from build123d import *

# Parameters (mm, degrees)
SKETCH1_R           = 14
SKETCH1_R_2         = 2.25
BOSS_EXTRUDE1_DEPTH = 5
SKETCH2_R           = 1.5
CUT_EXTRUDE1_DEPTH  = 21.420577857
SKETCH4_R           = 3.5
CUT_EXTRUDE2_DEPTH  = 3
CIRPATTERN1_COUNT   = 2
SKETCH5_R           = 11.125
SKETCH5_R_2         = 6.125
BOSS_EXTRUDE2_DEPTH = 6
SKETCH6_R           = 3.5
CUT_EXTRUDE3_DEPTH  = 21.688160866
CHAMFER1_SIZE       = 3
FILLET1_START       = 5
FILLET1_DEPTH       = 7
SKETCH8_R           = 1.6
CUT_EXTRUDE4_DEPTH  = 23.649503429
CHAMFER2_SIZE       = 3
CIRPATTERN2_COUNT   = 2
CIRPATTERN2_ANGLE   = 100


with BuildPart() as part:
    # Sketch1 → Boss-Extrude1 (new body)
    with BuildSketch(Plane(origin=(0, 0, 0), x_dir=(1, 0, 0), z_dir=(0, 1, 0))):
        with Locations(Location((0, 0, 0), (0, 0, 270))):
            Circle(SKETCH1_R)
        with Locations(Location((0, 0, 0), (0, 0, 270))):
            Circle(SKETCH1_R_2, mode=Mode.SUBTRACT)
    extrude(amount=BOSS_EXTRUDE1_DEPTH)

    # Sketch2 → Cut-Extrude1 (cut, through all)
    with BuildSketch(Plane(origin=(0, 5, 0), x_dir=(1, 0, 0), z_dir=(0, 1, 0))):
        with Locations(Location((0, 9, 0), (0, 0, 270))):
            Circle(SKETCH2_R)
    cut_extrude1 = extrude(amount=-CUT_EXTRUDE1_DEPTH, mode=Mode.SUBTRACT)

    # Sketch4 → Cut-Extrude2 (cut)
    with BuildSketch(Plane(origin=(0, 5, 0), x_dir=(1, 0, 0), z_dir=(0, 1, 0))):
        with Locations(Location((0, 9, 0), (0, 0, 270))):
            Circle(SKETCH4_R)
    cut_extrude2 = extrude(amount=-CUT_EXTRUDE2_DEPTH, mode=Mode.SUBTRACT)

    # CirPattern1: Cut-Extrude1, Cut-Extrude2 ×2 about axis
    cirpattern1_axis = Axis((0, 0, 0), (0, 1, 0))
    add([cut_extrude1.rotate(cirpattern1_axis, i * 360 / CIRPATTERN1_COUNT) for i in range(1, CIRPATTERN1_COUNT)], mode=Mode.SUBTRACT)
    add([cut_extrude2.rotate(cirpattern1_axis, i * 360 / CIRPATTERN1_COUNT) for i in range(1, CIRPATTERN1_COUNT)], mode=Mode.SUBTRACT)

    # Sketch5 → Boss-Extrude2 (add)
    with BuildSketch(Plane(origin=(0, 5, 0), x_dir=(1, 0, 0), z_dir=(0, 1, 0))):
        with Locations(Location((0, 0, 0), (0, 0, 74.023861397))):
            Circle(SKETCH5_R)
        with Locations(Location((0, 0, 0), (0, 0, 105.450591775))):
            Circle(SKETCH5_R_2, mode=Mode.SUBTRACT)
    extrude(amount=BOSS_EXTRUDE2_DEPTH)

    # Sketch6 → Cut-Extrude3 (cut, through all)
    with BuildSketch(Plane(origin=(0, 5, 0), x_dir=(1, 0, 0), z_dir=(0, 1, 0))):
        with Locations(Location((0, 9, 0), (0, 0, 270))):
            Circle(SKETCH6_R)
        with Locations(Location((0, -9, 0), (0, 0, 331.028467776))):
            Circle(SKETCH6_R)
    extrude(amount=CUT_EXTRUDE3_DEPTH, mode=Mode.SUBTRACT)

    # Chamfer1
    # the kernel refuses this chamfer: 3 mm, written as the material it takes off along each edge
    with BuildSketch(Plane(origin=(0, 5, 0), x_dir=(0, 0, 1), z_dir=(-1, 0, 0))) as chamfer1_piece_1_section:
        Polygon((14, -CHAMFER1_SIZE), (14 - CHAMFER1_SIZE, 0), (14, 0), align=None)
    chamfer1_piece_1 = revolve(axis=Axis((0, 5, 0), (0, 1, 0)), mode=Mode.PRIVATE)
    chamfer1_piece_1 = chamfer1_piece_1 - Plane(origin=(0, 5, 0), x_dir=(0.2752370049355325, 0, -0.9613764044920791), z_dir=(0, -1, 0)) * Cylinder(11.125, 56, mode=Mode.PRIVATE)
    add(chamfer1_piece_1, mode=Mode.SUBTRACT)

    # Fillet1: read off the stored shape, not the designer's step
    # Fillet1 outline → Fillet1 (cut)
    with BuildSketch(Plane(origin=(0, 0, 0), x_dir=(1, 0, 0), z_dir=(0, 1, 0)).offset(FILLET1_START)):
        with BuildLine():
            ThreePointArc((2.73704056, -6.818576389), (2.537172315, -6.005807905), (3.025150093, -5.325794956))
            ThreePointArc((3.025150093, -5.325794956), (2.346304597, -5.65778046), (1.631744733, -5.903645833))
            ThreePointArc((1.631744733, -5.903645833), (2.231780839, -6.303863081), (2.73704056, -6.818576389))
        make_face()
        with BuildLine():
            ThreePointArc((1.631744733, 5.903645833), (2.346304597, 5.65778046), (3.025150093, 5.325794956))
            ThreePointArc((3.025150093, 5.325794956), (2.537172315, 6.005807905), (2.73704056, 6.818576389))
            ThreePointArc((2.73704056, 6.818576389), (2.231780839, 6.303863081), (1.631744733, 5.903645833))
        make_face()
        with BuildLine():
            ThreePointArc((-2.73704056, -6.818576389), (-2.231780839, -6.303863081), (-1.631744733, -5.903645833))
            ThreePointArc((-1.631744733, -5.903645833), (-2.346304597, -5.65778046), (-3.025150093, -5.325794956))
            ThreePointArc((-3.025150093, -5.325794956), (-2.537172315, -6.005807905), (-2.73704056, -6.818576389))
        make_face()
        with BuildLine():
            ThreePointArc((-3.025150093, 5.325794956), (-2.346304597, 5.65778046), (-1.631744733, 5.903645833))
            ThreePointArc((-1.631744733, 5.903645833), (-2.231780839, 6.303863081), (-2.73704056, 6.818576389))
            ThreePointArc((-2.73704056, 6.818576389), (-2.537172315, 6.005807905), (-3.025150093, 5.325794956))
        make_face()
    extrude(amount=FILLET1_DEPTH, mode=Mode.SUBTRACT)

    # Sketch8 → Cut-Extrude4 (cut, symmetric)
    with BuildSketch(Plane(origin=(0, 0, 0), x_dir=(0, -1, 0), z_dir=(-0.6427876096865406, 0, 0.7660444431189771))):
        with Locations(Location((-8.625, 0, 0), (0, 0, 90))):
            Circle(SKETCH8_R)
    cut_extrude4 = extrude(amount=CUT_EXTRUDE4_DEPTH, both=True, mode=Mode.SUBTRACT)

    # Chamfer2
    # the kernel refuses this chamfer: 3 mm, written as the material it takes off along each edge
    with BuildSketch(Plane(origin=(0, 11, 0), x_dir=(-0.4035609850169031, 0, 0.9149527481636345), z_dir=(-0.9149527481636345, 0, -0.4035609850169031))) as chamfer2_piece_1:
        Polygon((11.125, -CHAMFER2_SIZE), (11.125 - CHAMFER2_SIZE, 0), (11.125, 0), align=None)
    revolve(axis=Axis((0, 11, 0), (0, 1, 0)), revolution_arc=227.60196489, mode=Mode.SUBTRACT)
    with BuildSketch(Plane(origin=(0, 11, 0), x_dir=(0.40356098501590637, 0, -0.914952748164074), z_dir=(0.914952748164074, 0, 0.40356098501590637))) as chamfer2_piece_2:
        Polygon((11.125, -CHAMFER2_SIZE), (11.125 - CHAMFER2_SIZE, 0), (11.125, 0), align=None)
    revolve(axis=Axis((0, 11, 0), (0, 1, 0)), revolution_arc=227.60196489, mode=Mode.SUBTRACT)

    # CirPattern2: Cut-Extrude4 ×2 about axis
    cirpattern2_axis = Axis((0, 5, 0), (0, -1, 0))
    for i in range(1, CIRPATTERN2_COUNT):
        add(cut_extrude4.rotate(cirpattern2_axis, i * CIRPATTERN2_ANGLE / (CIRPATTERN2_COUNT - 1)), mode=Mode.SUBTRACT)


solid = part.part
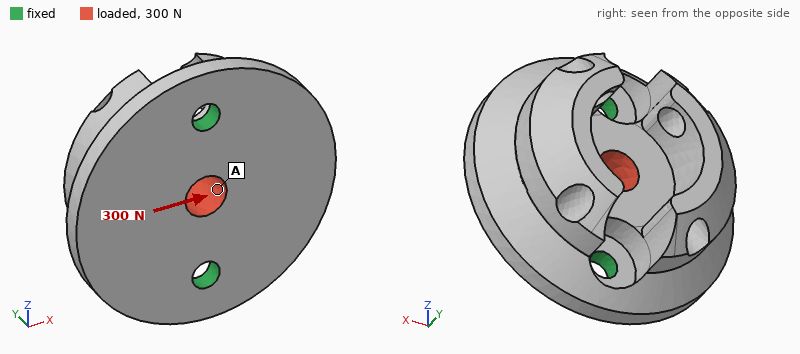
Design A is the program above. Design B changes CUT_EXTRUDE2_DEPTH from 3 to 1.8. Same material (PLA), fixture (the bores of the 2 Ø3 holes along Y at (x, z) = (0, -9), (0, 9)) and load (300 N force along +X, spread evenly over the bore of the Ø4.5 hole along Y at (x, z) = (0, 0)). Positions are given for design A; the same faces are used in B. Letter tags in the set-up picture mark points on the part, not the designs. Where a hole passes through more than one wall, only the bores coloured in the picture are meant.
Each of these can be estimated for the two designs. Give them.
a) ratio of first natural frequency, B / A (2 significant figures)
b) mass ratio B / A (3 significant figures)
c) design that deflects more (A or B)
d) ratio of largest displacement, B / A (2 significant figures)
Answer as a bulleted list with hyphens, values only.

- 1.5
- 1.02
- A
- 0.31
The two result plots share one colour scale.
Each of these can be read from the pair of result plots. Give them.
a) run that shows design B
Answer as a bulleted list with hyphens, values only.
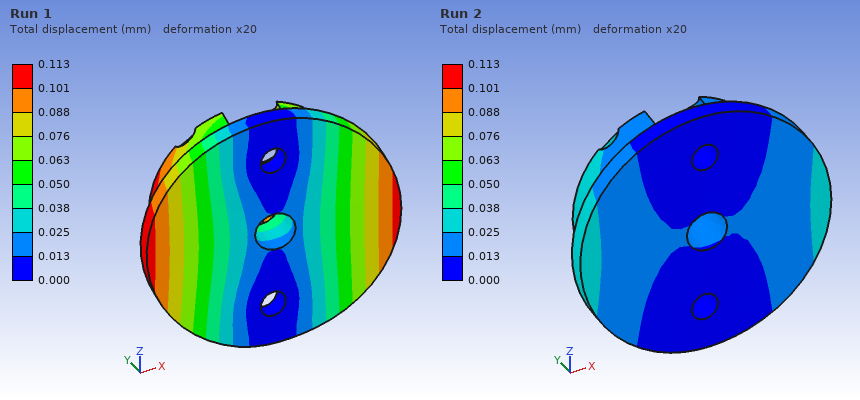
- Run 2
